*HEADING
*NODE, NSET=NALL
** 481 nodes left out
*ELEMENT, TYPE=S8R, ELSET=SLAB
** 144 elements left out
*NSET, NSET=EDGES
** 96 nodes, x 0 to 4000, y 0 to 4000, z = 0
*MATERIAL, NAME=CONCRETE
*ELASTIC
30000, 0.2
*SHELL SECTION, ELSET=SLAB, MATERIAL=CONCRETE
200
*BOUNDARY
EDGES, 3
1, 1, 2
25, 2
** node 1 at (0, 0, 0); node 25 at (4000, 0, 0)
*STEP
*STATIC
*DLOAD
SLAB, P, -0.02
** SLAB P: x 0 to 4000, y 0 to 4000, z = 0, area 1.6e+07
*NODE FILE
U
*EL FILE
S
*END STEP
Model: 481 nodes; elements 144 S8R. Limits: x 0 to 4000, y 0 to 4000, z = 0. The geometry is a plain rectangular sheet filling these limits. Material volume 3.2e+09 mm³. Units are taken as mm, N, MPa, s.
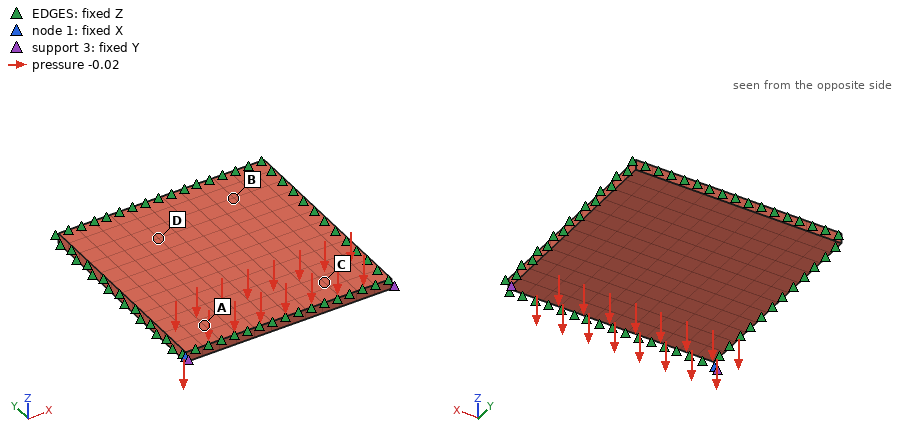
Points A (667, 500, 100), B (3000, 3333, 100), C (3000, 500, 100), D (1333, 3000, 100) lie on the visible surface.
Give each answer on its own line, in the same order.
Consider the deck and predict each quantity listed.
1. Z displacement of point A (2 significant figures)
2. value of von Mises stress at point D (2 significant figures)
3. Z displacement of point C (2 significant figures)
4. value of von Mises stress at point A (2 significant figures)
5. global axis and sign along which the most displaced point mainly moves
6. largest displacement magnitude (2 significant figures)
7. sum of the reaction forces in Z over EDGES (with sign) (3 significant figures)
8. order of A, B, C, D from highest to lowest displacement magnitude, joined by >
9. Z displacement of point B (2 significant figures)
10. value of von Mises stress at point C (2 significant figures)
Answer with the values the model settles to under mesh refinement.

-0.22 mm
1.8 MPa
-0.31 mm
2.4 MPa
-Z
1.1 mm
3.20e+05 N
D > B > C > A
-0.40 mm
2.0 MPa
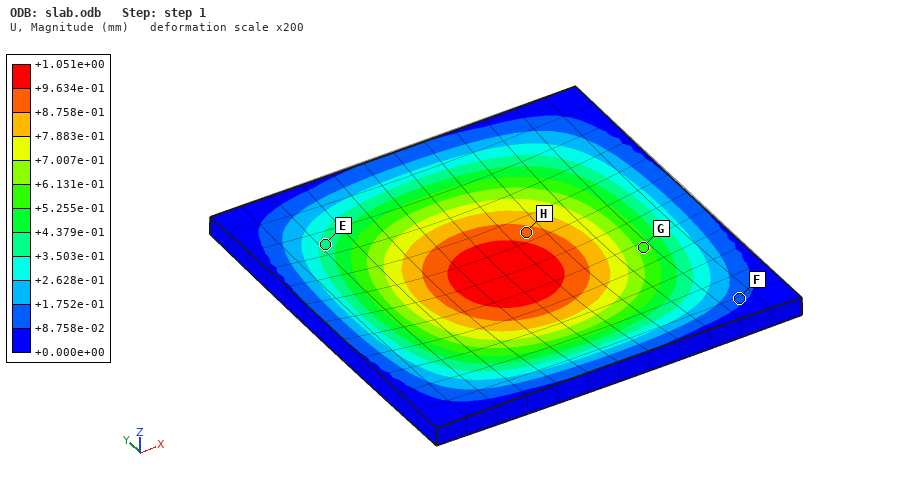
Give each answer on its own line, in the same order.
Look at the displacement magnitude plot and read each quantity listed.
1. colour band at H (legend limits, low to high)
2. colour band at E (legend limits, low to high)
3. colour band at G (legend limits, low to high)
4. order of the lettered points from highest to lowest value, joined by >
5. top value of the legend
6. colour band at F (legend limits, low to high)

+8.758e-01 to +9.634e-01 mm
+3.503e-01 to +4.379e-01 mm
+5.255e-01 to +6.131e-01 mm
H > G > E > F
+1.051e+00 mm
+8.758e-02 to +1.752e-01 mm
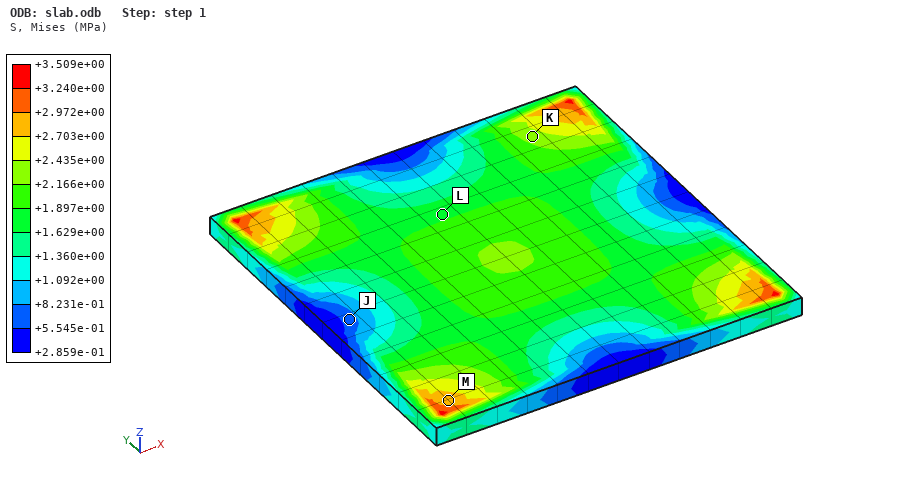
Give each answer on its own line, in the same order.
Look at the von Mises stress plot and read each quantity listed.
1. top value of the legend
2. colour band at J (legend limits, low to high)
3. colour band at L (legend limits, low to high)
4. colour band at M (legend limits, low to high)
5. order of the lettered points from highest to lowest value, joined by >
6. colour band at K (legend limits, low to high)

+3.509e+00 MPa
+5.545e-01 to +8.231e-01 MPa
+1.629e+00 to +1.897e+00 MPa
+2.703e+00 to +2.972e+00 MPa
M > K > L > J
+2.166e+00 to +2.435e+00 MPa
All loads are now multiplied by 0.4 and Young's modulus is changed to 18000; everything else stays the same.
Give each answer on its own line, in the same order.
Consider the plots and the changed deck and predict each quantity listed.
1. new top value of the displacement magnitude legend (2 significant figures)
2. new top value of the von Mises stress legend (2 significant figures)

0.70 mm
1.4 MPa
